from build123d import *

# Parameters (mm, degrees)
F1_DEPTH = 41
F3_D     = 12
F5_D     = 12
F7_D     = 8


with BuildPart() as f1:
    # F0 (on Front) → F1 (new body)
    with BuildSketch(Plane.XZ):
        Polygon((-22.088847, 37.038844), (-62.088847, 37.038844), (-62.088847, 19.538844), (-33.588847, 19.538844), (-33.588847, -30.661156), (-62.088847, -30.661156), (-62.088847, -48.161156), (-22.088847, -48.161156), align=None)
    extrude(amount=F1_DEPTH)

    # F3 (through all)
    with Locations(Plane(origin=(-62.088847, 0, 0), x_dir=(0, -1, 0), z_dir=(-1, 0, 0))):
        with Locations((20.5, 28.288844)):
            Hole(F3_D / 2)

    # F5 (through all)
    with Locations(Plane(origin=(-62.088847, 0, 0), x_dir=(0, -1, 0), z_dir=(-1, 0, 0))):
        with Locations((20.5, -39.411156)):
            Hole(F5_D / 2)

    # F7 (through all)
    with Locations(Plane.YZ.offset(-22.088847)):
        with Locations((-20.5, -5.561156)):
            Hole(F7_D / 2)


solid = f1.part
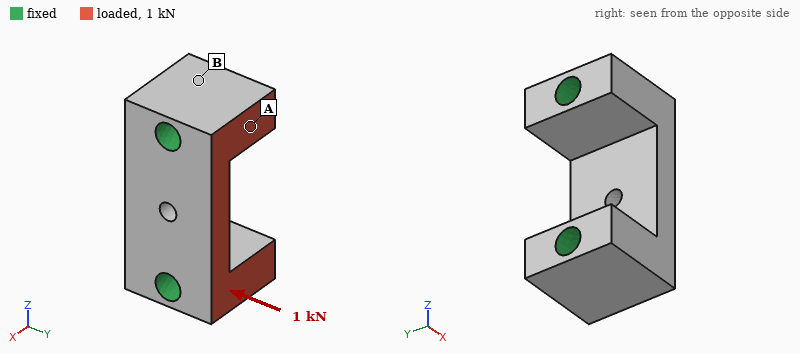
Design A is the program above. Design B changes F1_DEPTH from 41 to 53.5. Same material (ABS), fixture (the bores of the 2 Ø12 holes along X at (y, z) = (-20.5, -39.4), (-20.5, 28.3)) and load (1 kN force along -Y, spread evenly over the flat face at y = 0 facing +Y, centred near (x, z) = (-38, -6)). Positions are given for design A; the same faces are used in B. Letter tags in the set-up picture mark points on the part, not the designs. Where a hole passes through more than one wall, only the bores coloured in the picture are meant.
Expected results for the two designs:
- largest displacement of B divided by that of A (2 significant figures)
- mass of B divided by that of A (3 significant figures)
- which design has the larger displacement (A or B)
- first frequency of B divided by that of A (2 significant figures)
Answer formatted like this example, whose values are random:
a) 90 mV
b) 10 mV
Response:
a) 0.88
b) 1.35
c) A
d) 0.85
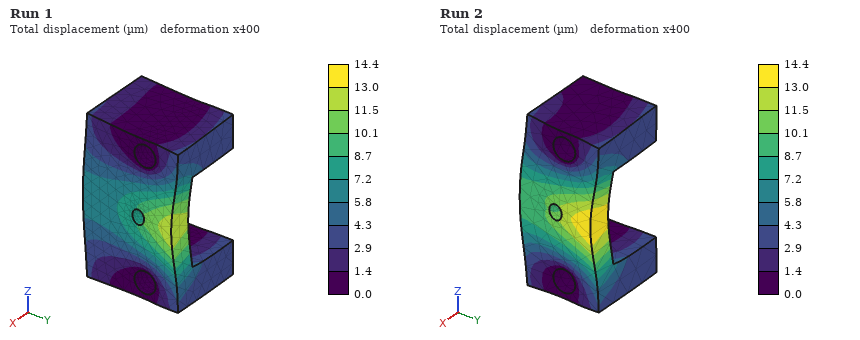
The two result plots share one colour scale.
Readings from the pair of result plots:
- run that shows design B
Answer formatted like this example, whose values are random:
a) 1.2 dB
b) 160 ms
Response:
a) Run 1
